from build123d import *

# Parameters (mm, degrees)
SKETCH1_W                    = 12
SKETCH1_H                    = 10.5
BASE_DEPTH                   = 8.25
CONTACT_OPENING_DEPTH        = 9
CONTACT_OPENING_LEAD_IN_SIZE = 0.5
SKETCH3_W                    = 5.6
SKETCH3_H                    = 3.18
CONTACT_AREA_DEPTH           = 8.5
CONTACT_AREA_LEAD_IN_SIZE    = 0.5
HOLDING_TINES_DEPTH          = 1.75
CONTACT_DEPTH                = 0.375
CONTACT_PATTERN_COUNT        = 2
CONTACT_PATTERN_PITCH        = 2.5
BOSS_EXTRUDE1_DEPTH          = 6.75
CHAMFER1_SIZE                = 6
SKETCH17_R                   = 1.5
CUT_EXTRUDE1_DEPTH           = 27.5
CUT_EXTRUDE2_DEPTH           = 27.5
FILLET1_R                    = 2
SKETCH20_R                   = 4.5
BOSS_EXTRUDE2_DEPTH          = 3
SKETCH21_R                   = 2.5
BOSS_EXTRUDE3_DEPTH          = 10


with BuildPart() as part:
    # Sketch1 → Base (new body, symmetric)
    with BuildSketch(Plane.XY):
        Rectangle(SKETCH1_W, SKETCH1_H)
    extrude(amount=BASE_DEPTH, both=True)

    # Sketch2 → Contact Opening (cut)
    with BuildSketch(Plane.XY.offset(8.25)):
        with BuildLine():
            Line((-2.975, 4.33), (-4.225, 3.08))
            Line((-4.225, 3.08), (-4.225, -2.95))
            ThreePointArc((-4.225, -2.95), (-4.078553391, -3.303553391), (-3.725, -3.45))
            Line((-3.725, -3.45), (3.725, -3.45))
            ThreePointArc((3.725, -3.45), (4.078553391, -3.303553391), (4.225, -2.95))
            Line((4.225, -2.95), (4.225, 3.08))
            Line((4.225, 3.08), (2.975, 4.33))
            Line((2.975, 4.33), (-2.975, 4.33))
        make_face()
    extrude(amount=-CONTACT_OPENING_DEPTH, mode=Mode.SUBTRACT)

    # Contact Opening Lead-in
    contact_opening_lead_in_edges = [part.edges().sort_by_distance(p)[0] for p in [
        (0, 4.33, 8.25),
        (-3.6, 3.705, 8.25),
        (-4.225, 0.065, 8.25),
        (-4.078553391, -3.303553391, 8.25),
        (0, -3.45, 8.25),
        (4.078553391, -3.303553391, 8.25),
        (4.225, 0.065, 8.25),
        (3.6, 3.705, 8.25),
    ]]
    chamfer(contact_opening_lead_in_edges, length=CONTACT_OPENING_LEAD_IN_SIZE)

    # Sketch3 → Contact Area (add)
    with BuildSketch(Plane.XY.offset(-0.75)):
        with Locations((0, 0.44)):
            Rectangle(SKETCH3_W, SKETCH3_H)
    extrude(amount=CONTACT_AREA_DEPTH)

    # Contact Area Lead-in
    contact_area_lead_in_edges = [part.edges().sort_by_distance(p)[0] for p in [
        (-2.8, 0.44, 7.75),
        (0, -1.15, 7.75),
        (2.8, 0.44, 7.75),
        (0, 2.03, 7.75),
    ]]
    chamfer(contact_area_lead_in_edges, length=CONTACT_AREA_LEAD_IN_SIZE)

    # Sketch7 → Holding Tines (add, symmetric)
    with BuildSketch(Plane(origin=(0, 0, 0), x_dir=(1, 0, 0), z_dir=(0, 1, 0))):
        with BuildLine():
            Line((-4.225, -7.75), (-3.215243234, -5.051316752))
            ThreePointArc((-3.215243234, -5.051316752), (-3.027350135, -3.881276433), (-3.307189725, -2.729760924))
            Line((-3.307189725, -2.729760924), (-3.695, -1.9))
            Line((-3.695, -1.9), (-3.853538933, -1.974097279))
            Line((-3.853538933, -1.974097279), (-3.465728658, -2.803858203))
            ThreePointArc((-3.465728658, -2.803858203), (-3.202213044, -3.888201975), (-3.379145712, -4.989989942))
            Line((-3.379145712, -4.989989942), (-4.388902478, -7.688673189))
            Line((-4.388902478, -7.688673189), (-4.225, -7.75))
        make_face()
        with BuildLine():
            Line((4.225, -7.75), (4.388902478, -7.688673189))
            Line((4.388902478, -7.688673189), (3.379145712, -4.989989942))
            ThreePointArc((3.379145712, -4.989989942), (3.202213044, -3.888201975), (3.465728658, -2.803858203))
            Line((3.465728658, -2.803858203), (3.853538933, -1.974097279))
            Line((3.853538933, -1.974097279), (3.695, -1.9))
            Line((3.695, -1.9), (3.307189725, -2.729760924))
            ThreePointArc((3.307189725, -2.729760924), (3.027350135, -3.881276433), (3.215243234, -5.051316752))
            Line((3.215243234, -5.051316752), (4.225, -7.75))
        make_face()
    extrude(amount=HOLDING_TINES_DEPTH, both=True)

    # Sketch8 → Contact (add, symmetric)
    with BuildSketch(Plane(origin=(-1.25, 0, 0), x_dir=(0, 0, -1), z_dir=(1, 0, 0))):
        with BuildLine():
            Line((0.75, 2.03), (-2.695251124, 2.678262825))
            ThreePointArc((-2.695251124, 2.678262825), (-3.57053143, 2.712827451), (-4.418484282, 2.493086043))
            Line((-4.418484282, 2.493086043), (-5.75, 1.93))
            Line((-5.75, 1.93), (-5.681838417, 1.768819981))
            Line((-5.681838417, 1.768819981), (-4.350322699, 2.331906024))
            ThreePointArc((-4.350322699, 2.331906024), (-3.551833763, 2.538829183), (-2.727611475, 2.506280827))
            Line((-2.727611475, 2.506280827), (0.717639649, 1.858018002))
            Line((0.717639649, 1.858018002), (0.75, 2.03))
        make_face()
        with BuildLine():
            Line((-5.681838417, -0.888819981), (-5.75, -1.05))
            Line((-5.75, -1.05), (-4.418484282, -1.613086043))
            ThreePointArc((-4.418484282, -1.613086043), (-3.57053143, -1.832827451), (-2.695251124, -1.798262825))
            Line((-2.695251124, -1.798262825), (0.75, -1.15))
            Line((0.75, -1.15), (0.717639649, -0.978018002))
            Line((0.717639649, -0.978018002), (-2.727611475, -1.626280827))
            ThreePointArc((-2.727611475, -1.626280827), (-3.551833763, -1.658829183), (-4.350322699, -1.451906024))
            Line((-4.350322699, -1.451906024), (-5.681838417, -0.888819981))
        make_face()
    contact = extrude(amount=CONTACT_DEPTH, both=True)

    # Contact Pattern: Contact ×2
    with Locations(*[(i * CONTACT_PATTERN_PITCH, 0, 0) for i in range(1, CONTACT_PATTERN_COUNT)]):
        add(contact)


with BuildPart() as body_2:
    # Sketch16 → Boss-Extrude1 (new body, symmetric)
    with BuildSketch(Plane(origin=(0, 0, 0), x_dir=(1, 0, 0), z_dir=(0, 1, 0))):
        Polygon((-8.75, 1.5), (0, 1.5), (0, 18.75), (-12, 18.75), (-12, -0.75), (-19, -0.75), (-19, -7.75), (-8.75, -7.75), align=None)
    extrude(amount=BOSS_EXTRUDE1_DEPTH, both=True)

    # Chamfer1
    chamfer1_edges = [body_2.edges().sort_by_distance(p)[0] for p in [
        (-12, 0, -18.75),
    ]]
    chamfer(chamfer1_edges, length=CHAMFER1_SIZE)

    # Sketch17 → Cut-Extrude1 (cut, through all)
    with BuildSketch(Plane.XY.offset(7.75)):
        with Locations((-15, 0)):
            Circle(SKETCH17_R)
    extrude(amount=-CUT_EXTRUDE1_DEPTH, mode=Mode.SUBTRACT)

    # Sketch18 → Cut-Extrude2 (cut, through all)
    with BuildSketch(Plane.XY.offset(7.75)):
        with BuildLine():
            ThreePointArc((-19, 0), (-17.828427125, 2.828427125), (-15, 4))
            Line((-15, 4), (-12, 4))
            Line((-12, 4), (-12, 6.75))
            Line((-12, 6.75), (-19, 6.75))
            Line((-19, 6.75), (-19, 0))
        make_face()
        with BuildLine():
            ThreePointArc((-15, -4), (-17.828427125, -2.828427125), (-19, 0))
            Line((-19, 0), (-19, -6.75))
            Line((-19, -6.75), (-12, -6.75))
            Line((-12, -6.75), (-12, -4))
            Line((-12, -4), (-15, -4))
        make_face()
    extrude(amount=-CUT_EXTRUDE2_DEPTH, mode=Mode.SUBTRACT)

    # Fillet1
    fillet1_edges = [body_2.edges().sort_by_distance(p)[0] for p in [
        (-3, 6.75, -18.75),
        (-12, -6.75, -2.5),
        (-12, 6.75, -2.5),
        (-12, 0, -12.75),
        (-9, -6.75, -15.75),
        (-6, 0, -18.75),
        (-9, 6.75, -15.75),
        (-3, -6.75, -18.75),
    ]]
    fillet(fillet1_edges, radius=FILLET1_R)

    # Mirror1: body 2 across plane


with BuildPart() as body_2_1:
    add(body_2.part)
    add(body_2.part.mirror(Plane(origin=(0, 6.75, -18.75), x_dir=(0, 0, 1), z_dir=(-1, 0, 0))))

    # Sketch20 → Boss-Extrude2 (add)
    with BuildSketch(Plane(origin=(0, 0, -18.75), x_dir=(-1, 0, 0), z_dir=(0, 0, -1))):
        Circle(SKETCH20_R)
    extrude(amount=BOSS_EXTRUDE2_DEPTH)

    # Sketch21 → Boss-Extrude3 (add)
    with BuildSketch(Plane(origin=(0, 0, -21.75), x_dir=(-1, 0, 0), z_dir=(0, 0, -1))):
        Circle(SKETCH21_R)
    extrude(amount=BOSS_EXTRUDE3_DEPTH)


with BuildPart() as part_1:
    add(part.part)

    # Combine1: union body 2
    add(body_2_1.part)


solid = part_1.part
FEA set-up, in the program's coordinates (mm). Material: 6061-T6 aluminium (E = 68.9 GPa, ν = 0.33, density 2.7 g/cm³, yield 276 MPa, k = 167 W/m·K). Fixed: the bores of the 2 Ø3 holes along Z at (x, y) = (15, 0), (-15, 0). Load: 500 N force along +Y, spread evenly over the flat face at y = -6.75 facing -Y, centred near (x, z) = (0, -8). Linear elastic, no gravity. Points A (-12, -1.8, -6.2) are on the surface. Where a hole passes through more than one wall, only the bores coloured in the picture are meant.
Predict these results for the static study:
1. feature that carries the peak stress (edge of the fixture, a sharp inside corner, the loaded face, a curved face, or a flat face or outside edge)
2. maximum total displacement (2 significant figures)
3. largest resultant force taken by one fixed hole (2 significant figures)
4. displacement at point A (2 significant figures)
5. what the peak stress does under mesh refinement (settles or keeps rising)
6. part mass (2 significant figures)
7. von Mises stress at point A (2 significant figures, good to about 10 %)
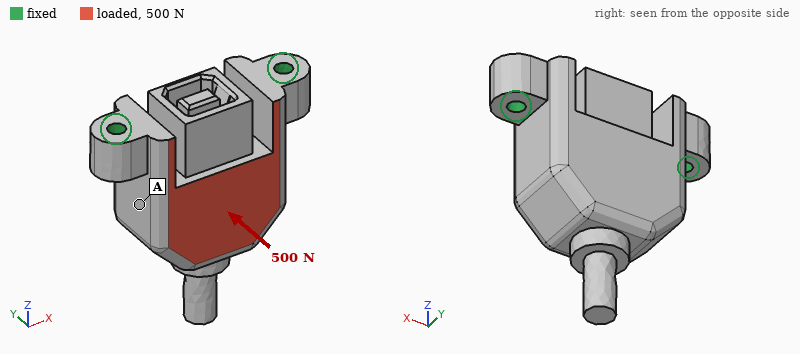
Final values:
edge of the fixture
49 µm
250 N
14 µm
keeps rising
20 g
8.5 MPa
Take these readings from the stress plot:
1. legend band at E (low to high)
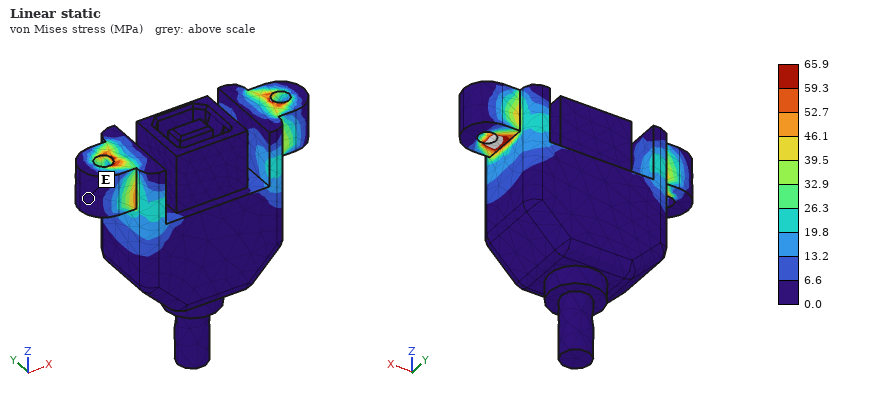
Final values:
0.0 to 6.6 MPa
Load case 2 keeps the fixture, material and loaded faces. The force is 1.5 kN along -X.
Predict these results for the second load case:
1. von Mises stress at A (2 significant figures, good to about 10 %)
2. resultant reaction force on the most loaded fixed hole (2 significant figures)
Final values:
11 MPa
1.0 kN
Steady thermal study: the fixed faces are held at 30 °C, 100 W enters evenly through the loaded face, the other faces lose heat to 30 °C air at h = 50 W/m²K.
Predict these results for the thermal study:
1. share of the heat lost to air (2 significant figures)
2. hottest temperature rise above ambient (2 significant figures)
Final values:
8.3 %
74 K
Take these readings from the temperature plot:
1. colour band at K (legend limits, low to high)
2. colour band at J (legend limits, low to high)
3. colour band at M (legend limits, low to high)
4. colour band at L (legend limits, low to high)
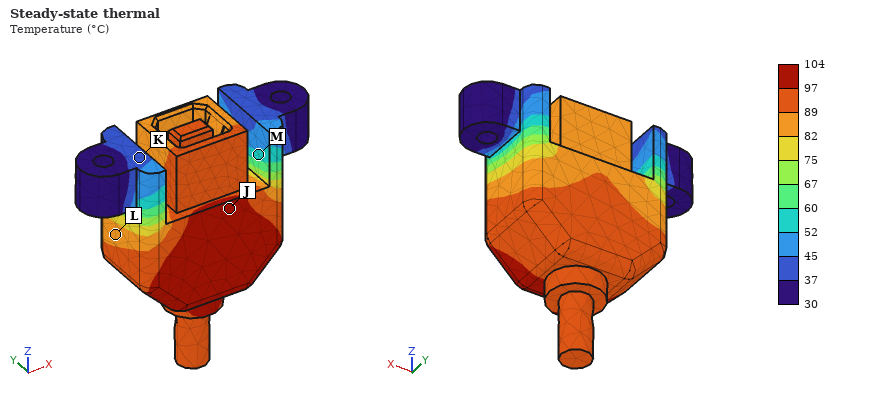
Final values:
37 to 45 °C
97 to 104 °C
52 to 60 °C
82 to 89 °C
